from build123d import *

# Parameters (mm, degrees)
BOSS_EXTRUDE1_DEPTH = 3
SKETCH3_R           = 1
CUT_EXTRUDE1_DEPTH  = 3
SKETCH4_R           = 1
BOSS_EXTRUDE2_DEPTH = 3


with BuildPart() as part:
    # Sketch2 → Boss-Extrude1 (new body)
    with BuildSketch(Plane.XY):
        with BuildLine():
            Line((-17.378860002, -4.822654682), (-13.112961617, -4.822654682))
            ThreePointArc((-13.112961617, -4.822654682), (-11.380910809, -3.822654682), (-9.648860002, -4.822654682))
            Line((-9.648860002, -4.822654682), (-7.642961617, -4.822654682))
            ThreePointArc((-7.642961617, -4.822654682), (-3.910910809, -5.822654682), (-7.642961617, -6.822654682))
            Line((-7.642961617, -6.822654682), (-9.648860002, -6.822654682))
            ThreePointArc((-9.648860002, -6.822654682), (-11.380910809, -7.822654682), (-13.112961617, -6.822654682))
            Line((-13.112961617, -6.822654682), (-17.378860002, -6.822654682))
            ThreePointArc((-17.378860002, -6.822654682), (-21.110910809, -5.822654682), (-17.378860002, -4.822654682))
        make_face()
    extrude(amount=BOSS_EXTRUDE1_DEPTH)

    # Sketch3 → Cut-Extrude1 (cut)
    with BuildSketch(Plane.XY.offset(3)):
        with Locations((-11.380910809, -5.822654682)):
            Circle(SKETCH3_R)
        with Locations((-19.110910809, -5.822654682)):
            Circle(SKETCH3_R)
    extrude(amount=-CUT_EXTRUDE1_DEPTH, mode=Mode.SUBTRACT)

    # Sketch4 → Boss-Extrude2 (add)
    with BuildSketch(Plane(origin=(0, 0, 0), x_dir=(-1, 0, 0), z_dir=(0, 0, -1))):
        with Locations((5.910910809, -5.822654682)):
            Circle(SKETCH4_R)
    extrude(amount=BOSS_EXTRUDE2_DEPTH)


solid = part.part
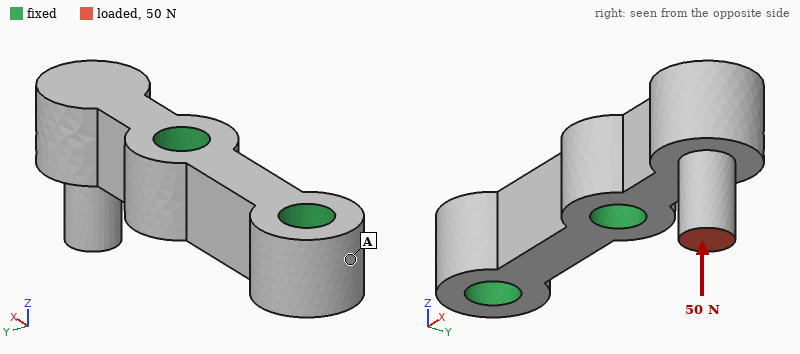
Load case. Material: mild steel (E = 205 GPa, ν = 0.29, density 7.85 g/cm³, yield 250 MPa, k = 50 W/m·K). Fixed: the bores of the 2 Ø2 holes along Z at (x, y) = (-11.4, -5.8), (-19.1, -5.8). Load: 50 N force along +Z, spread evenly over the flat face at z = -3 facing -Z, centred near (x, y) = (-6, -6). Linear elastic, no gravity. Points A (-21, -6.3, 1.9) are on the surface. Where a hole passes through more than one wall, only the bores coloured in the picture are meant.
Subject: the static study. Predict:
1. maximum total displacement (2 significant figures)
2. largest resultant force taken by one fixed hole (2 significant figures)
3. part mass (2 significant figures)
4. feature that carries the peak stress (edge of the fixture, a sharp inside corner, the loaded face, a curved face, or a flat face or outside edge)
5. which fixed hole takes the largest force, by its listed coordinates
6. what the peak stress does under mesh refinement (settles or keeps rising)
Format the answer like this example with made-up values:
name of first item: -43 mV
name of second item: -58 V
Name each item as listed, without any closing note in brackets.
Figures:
maximum total displacement: 3.9 µm
largest resultant force taken by one fixed hole: 50 N
part mass: 1.1 g
feature that carries the peak stress: edge of the fixture
which fixed hole takes the largest force, by its listed coordinates: (-11.4, -5.8)
what the peak stress does under mesh refinement: keeps rising
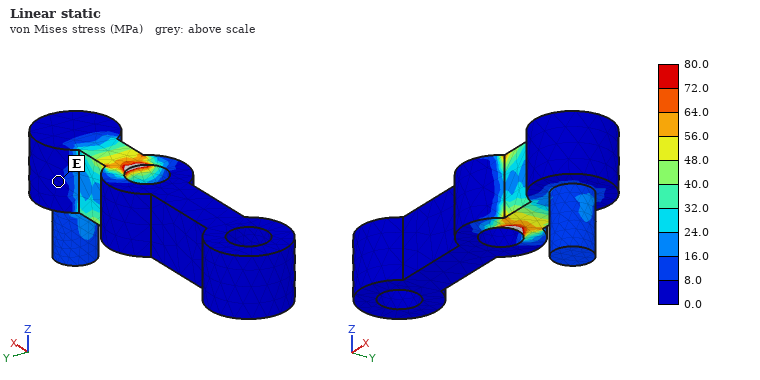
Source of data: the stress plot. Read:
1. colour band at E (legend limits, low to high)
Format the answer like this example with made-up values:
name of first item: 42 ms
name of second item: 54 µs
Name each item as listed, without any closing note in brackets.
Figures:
colour band at E: 0.0 to 8.0 MPa
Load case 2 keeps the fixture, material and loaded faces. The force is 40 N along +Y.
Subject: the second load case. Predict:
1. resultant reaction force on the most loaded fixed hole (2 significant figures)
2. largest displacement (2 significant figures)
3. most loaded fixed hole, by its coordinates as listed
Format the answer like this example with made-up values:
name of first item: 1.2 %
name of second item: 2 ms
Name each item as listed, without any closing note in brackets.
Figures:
resultant reaction force on the most loaded fixed hole: 41 N
largest displacement: 14 µm
most loaded fixed hole, by its coordinates as listed: (-11.4, -5.8)
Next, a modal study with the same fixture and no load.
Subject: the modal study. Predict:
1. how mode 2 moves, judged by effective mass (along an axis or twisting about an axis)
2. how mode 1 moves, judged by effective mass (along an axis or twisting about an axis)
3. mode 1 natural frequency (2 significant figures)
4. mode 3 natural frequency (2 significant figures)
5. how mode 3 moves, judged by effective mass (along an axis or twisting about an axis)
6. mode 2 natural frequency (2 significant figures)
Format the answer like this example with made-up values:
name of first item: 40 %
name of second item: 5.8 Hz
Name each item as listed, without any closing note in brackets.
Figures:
how mode 2 moves, judged by effective mass: along Z
how mode 1 moves, judged by effective mass: along Y
mode 1 natural frequency: 27 kHz
mode 3 natural frequency: 51 kHz
how mode 3 moves, judged by effective mass: twisting about X
mode 2 natural frequency: 36 kHz
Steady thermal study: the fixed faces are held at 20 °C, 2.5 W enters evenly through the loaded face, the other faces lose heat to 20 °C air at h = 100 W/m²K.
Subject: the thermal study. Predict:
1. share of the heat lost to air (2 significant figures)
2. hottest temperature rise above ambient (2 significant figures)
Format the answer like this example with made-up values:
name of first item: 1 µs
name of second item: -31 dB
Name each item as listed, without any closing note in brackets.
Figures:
share of the heat lost to air: 11 %
hottest temperature rise above ambient: 82 K
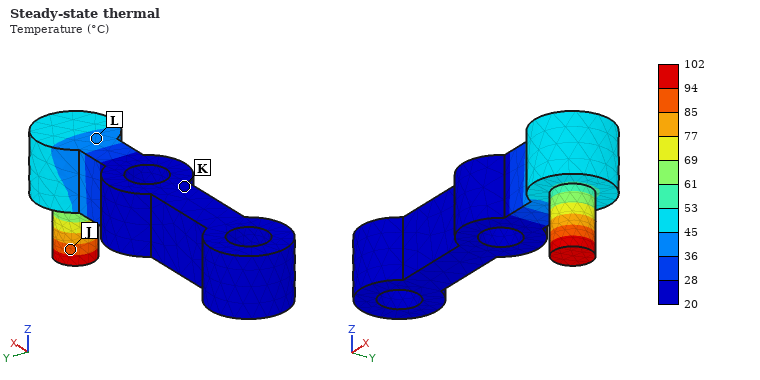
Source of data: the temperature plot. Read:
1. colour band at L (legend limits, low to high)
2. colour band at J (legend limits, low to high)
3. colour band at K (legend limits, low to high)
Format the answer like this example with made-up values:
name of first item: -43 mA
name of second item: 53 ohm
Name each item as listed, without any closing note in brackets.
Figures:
colour band at L: 36 to 45 °C
colour band at J: 85 to 94 °C
colour band at K: 20 to 28 °C
